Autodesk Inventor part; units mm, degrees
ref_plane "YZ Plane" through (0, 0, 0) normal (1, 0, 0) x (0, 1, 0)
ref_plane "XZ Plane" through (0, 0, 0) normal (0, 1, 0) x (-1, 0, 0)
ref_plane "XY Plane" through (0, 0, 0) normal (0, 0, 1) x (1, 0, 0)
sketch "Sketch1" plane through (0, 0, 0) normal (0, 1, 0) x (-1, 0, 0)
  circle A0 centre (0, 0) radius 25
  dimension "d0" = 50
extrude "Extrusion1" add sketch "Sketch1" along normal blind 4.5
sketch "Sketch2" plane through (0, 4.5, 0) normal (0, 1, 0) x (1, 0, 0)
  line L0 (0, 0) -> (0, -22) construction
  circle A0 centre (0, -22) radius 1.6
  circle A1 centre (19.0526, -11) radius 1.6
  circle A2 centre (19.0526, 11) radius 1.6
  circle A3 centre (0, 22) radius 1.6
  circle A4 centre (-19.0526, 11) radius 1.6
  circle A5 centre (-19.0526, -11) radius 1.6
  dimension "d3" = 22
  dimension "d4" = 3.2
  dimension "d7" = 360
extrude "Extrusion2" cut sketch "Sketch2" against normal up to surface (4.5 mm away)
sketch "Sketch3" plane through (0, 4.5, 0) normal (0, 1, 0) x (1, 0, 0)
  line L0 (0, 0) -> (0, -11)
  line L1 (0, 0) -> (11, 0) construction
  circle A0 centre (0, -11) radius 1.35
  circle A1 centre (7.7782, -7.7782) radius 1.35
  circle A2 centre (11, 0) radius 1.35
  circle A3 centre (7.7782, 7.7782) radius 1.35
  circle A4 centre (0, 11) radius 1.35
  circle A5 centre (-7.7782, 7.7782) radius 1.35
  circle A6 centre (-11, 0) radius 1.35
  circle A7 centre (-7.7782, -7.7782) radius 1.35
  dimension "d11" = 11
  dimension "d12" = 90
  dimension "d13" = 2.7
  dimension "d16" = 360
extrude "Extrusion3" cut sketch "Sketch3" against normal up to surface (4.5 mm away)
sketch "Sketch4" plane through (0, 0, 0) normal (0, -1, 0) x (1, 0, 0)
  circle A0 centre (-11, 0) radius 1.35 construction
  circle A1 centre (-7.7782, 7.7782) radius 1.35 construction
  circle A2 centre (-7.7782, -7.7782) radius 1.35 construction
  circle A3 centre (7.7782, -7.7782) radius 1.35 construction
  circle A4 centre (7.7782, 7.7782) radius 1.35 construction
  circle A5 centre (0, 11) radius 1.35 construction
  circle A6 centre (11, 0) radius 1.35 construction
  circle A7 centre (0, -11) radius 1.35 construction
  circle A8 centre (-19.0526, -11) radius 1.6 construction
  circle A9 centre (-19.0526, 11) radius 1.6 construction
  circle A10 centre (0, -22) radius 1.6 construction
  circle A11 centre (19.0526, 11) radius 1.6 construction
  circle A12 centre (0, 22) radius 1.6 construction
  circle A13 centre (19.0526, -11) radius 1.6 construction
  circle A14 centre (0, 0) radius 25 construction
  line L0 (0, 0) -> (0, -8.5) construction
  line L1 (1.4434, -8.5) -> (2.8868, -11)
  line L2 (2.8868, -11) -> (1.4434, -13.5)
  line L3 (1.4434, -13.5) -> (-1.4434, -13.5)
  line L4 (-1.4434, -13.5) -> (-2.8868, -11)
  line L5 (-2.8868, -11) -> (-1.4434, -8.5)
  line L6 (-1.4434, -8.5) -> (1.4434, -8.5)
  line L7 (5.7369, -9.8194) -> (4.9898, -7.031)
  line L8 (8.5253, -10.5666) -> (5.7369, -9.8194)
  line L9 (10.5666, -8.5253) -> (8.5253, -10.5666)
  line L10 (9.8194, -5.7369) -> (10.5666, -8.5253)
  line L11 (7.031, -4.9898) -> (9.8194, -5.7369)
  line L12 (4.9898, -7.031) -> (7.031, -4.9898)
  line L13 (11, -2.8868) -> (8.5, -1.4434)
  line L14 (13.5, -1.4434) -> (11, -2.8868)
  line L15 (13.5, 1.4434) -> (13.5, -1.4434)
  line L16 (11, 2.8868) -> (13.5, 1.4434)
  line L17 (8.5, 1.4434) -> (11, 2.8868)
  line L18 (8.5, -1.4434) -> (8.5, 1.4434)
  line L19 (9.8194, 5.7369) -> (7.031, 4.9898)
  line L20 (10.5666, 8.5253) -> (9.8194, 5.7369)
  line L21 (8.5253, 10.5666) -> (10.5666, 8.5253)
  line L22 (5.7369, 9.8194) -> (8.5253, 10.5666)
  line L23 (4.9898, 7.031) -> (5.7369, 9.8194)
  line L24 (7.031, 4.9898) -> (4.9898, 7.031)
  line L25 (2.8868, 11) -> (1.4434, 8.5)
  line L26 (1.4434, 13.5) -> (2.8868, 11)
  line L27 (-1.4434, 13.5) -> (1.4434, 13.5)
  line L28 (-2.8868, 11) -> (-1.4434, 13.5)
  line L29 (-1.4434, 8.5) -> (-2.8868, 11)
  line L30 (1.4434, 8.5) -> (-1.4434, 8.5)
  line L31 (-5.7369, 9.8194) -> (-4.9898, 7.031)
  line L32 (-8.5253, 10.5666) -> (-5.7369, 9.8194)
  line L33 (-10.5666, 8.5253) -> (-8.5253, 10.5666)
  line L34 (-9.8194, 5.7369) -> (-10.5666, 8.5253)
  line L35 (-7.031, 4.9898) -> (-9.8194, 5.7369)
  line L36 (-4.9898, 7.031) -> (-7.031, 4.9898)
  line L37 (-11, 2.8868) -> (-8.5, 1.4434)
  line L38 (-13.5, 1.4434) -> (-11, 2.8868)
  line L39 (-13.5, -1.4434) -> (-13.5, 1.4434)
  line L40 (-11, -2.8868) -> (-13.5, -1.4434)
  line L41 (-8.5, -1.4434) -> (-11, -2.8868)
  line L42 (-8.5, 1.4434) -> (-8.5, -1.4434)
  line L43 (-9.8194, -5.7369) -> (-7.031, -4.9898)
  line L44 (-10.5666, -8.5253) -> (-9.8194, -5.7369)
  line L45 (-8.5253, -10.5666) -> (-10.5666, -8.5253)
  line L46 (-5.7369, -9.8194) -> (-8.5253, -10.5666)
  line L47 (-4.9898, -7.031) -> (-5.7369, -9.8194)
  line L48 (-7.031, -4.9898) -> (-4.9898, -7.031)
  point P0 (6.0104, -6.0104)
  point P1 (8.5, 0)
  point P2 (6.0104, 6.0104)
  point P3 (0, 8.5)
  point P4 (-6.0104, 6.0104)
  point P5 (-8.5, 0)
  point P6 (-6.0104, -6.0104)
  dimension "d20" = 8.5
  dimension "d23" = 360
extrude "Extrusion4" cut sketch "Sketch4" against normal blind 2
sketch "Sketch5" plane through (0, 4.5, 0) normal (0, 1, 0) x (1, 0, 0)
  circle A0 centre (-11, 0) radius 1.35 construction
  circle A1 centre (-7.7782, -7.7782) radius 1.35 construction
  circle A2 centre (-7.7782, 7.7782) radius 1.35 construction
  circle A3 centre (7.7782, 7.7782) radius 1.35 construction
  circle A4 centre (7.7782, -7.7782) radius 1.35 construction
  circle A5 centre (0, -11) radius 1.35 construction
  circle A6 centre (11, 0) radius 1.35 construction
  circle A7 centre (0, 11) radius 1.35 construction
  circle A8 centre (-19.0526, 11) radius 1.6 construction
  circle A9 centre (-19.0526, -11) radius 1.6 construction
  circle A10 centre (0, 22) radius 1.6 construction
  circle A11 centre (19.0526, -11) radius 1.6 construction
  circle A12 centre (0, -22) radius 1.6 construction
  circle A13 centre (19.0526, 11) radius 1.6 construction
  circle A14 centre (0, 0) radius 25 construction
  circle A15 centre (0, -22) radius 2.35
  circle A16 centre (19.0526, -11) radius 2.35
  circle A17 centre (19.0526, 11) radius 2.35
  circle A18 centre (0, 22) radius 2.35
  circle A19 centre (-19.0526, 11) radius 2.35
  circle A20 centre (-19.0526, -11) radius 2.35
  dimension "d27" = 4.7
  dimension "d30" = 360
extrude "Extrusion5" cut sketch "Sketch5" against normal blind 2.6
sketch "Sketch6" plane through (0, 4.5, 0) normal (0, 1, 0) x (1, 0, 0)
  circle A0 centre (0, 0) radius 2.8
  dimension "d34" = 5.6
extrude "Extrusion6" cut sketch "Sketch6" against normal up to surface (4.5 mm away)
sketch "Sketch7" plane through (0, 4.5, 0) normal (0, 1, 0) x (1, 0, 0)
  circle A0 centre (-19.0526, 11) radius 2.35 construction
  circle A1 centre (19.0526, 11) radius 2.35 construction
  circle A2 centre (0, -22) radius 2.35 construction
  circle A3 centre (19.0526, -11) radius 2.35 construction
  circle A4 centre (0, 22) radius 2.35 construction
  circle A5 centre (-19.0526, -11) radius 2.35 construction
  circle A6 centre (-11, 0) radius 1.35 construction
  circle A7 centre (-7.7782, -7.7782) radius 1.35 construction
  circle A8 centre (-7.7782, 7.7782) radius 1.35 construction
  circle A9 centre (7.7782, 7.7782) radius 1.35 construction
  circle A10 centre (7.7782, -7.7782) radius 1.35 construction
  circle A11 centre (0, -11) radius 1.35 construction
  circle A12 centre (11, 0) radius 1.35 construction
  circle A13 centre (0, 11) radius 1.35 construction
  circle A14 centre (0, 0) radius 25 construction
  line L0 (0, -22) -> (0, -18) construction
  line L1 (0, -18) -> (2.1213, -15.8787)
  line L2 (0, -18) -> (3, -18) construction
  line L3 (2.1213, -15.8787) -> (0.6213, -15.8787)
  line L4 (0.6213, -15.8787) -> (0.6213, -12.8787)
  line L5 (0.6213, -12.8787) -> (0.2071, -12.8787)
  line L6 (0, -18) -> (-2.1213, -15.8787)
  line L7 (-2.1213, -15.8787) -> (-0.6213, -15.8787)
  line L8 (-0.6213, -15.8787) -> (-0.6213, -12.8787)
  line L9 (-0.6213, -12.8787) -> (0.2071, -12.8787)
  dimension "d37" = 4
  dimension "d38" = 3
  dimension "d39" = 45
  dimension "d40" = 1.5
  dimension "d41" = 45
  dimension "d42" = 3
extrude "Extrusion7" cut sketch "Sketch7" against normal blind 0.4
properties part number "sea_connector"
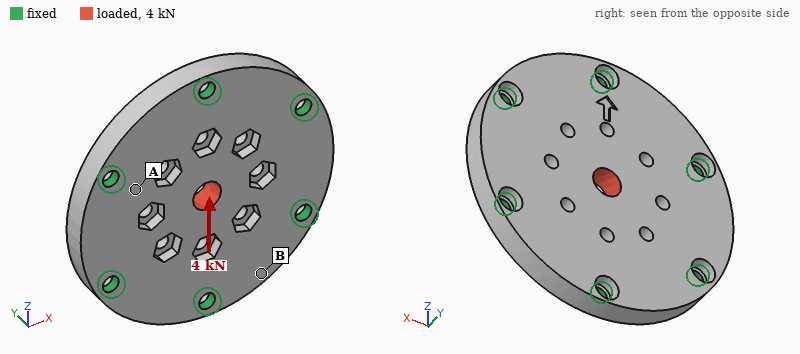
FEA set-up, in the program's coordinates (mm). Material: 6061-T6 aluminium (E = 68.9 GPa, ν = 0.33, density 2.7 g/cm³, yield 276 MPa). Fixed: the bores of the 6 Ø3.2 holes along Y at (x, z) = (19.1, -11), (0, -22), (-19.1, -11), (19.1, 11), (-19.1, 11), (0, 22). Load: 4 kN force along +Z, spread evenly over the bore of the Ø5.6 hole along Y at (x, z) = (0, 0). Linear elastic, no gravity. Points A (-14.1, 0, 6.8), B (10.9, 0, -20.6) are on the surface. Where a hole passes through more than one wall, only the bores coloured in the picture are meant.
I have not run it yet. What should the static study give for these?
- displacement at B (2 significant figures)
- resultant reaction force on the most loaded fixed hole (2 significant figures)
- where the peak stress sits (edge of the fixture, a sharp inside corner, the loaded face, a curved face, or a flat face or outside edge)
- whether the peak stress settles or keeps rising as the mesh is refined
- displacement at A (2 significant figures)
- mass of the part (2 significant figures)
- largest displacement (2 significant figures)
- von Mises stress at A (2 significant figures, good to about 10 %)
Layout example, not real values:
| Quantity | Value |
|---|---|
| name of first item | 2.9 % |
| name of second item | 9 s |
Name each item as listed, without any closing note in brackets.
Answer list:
| Quantity | Value |
|---|---|
| displacement at B | 3.1 µm |
| resultant reaction force on the most loaded fixed hole | 930 N |
| where the peak stress sits | edge of the fixture |
| whether the peak stress settles or keeps rising as the mesh is refined | keeps rising |
| displacement at A | 2.9 µm |
| mass of the part | 21 g |
| largest displacement | 13 µm |
| von Mises stress at A | 23 MPa |
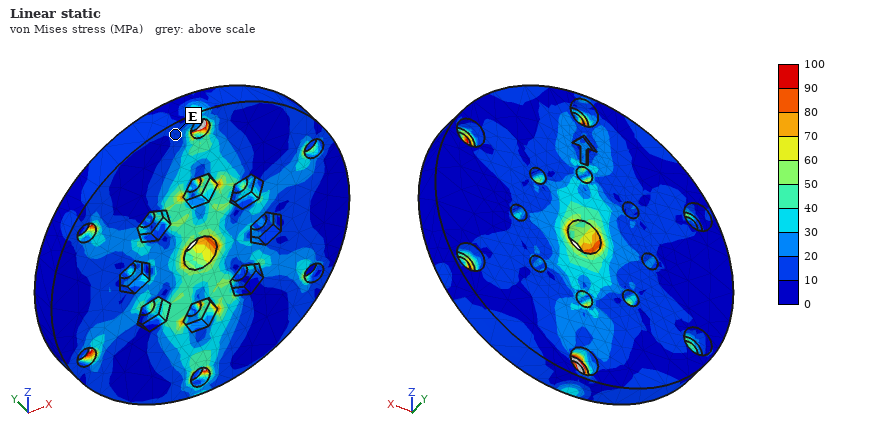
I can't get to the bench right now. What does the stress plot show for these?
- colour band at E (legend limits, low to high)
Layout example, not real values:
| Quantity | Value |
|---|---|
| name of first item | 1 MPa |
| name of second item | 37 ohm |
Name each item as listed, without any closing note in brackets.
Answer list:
| Quantity | Value |
|---|---|
| colour band at E | 10 to 20 MPa |
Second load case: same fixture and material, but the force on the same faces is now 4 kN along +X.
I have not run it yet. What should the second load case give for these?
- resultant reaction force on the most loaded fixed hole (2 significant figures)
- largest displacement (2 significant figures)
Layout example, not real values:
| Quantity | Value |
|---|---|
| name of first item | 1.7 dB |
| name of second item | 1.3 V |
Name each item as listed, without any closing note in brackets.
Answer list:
| Quantity | Value |
|---|---|
| resultant reaction force on the most loaded fixed hole | 830 N |
| largest displacement | 12 µm |
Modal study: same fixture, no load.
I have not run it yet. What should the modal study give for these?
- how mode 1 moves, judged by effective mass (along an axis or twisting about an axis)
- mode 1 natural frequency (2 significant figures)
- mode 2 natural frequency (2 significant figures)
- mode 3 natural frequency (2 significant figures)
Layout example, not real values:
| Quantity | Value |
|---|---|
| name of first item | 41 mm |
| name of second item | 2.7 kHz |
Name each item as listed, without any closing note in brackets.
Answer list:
| Quantity | Value |
|---|---|
| how mode 1 moves, judged by effective mass | along Y |
| mode 1 natural frequency | 15 kHz |
| mode 2 natural frequency | 27 kHz |
| mode 3 natural frequency | 28 kHz |
